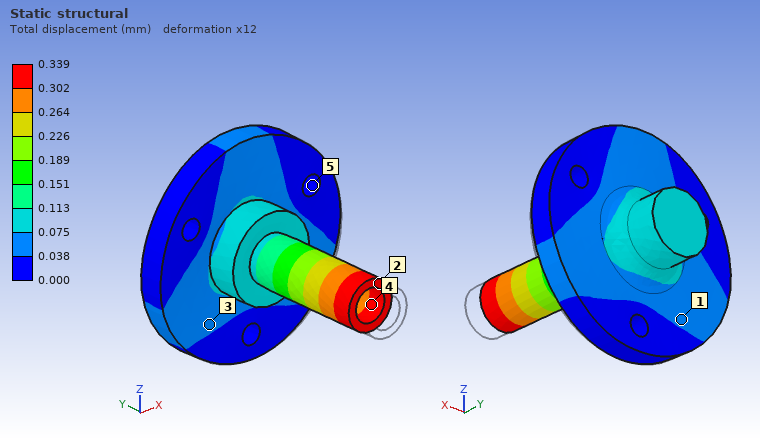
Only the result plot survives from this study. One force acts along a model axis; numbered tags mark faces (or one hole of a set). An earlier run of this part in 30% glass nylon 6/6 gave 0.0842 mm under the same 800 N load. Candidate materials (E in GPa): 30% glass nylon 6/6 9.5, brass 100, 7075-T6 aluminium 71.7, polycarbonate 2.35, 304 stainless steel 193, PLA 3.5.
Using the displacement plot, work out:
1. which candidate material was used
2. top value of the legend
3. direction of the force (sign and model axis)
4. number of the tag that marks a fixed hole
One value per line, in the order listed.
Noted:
polycarbonate
0.339 mm
+Y
5
